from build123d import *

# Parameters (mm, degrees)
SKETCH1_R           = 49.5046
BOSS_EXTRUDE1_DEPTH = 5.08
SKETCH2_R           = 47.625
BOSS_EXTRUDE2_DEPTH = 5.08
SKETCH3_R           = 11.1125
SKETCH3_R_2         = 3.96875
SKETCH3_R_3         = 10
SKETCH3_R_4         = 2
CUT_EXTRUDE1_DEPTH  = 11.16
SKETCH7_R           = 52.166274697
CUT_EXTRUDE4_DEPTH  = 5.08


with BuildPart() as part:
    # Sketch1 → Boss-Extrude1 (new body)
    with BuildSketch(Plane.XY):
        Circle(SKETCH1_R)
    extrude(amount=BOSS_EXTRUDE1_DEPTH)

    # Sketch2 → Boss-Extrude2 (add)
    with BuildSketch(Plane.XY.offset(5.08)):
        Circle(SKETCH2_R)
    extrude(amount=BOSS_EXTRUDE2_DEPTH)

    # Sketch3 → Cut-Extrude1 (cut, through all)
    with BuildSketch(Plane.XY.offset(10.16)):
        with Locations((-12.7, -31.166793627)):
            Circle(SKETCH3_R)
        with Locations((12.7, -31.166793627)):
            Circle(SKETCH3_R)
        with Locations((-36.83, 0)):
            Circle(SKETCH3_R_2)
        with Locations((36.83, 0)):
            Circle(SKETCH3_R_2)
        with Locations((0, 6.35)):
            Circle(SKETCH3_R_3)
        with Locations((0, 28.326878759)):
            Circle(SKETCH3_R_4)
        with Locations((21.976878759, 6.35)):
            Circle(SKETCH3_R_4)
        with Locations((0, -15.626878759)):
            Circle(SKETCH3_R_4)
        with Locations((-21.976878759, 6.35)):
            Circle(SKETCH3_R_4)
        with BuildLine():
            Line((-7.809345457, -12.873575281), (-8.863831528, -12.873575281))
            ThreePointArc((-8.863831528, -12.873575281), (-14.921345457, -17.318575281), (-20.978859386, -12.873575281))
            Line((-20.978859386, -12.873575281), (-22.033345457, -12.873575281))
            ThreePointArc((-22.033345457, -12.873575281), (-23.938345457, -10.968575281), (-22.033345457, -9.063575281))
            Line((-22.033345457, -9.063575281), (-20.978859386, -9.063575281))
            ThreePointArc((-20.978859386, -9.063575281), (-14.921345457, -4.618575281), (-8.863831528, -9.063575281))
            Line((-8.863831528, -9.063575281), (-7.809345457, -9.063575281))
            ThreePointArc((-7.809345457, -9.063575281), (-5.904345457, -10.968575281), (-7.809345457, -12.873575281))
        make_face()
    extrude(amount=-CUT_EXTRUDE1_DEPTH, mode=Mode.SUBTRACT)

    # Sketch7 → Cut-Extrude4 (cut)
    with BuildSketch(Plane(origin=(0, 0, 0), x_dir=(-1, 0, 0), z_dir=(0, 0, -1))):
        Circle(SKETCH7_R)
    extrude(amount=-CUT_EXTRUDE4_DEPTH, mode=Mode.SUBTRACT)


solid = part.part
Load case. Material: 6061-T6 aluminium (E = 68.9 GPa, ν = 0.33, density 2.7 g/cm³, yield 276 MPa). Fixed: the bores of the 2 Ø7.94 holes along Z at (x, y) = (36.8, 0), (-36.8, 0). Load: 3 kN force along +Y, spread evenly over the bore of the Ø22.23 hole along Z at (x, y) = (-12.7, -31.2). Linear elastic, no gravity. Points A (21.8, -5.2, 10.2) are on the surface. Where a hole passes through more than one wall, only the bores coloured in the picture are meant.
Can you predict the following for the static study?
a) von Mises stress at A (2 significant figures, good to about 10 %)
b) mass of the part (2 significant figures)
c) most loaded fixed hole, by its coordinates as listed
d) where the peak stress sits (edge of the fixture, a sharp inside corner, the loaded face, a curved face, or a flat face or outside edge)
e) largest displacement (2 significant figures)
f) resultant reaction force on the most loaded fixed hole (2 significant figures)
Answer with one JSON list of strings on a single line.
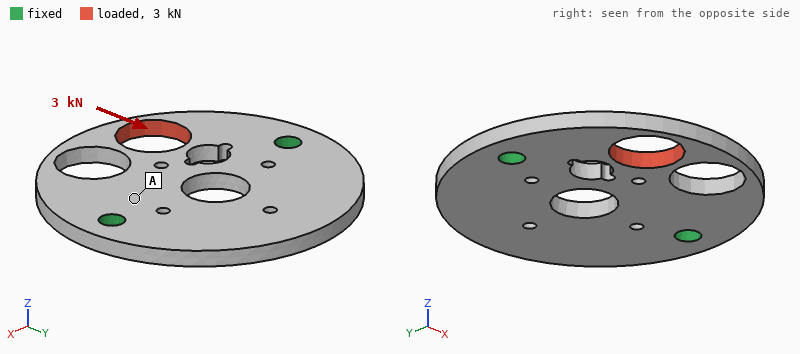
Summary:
["9.5 MPa", "79 g", "(-36.8, 0)", "a curved face", "33 µm", "2.1 kN"]
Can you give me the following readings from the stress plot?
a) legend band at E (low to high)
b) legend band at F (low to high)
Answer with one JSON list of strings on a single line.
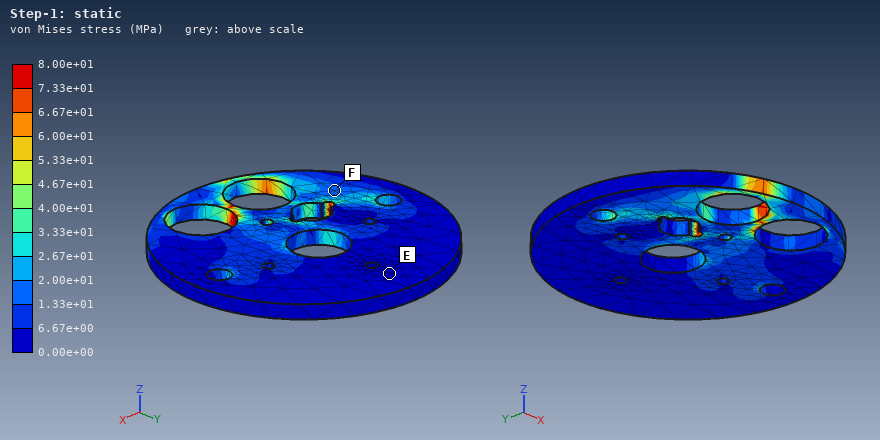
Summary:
["0.00e+00 to 6.67e+00 MPa", "1.33e+01 to 2.00e+01 MPa"]
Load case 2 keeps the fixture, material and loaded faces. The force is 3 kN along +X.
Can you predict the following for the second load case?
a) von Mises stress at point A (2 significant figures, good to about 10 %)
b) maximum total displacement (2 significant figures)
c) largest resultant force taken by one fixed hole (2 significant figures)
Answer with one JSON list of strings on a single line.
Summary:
["17 MPa", "58 µm", "1.9 kN"]
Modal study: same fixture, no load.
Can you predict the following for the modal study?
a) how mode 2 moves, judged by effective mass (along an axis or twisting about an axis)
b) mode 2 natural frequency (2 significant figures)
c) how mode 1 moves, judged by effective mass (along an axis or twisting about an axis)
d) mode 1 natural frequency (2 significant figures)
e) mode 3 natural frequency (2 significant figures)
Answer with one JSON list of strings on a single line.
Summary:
["along Z", "2400 Hz", "along Z", "1900 Hz", "4700 Hz"]
